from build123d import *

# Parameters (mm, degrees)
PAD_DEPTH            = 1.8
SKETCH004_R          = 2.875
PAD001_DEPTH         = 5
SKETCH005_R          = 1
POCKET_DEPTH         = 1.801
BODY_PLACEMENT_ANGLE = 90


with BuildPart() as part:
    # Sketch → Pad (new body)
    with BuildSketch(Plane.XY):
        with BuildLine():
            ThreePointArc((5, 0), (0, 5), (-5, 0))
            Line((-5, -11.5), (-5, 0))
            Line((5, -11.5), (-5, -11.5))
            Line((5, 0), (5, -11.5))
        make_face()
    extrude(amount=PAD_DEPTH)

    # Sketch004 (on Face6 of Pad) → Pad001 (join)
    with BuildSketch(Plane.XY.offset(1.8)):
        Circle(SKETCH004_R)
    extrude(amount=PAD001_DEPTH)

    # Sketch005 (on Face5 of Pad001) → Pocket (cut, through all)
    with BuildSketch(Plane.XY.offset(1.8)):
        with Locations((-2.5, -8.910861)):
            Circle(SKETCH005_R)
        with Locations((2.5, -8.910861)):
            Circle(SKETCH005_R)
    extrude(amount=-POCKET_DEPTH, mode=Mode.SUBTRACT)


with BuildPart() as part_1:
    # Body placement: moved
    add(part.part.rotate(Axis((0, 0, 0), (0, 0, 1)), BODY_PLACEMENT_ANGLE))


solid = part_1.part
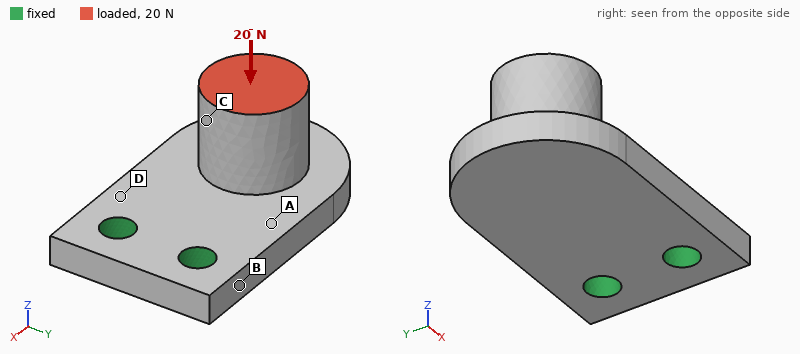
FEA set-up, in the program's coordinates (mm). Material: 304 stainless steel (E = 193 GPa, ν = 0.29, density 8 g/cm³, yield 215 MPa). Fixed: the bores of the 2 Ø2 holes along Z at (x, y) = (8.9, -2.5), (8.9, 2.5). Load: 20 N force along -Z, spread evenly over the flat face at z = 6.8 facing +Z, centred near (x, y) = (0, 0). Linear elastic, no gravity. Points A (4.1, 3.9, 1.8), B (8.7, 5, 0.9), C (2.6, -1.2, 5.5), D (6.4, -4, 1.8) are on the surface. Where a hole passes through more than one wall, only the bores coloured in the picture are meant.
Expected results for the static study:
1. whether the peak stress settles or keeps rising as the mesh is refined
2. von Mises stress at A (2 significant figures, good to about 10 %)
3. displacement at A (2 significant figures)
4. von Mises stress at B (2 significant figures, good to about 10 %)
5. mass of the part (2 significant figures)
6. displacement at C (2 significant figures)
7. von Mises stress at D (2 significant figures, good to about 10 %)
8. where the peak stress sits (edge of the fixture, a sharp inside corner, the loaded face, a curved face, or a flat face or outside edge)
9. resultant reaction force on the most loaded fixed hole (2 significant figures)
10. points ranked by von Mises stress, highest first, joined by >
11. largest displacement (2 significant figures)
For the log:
keeps rising
15 MPa
1.5 µm
7.7 MPa
3.2 g
4.0 µm
22 MPa
edge of the fixture
10 N
D > A > B > C
7.8 µm
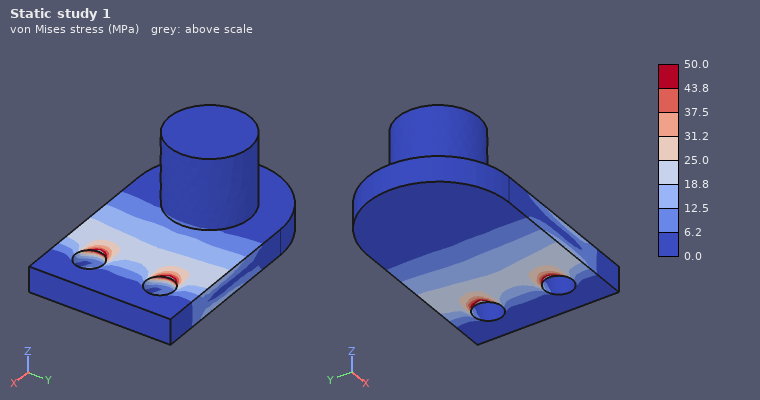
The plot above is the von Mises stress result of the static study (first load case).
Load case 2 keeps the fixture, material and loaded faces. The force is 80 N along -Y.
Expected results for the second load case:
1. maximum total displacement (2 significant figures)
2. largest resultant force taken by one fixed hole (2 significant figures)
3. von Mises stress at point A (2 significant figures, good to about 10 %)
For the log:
12 µm
130 N
46 MPa
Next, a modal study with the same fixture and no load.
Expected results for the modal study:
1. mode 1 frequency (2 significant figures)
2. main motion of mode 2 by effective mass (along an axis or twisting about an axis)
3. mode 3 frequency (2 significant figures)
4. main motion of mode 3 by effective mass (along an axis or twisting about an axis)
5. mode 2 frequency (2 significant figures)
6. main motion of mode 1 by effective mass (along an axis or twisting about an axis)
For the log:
6500 Hz
along Y
31 kHz
along Y
17 kHz
along Z
